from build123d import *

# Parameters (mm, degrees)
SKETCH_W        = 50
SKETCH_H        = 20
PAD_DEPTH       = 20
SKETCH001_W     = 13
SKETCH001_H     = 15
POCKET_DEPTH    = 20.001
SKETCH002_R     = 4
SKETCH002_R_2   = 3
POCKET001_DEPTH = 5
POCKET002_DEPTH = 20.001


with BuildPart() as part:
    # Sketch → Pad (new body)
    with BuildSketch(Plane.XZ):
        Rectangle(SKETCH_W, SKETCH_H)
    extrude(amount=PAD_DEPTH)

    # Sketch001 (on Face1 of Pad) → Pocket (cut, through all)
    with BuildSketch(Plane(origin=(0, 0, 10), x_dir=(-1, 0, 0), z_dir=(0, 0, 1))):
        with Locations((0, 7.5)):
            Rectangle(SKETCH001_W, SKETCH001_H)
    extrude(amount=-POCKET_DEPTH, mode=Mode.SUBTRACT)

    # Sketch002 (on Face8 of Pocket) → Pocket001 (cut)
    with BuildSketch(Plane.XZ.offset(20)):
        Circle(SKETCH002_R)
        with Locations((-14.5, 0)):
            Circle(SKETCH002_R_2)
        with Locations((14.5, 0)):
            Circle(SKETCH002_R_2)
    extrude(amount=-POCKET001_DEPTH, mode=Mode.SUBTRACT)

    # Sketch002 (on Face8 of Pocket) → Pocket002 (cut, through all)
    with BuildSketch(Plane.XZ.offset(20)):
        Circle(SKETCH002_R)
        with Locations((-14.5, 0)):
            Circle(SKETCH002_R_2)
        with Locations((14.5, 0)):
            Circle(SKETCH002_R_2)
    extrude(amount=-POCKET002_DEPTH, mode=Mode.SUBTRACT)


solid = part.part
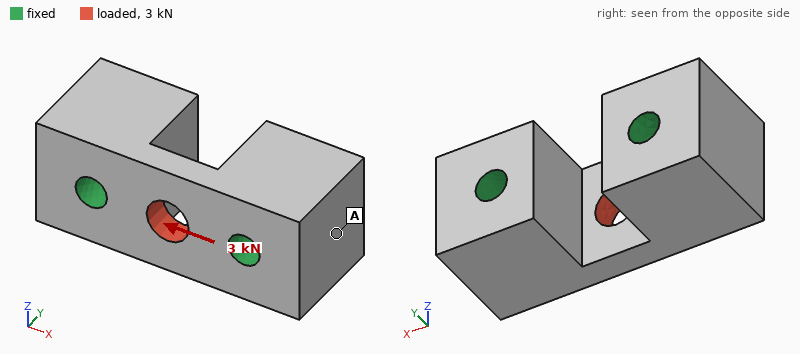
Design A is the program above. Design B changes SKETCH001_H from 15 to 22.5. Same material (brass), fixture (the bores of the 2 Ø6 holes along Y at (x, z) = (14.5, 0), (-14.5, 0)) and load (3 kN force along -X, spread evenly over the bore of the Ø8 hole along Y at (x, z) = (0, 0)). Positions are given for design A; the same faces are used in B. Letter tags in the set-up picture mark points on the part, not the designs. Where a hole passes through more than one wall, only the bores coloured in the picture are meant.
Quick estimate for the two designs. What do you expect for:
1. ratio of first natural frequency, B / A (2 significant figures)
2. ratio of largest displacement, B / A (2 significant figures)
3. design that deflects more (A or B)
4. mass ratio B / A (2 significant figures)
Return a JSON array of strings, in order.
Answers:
["0.88", "3.4", "B", "0.95"]
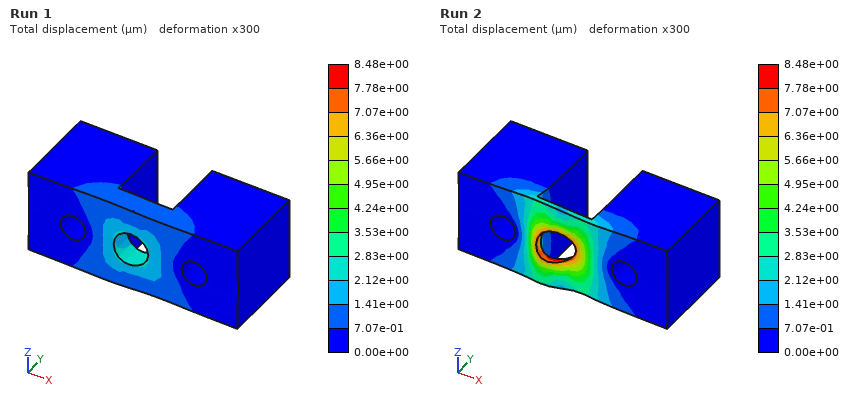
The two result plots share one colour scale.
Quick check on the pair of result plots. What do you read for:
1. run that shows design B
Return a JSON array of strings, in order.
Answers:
["Run 2"]
